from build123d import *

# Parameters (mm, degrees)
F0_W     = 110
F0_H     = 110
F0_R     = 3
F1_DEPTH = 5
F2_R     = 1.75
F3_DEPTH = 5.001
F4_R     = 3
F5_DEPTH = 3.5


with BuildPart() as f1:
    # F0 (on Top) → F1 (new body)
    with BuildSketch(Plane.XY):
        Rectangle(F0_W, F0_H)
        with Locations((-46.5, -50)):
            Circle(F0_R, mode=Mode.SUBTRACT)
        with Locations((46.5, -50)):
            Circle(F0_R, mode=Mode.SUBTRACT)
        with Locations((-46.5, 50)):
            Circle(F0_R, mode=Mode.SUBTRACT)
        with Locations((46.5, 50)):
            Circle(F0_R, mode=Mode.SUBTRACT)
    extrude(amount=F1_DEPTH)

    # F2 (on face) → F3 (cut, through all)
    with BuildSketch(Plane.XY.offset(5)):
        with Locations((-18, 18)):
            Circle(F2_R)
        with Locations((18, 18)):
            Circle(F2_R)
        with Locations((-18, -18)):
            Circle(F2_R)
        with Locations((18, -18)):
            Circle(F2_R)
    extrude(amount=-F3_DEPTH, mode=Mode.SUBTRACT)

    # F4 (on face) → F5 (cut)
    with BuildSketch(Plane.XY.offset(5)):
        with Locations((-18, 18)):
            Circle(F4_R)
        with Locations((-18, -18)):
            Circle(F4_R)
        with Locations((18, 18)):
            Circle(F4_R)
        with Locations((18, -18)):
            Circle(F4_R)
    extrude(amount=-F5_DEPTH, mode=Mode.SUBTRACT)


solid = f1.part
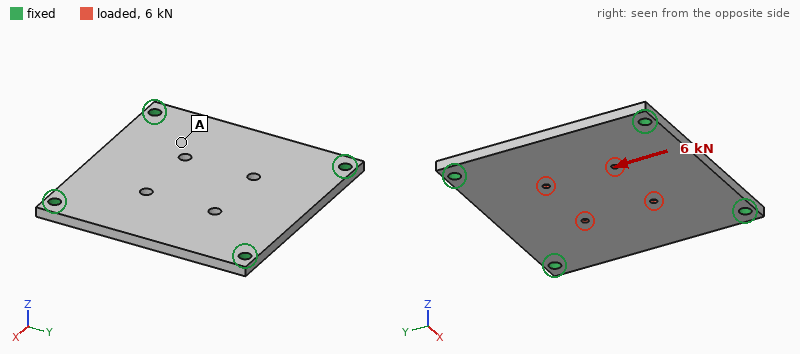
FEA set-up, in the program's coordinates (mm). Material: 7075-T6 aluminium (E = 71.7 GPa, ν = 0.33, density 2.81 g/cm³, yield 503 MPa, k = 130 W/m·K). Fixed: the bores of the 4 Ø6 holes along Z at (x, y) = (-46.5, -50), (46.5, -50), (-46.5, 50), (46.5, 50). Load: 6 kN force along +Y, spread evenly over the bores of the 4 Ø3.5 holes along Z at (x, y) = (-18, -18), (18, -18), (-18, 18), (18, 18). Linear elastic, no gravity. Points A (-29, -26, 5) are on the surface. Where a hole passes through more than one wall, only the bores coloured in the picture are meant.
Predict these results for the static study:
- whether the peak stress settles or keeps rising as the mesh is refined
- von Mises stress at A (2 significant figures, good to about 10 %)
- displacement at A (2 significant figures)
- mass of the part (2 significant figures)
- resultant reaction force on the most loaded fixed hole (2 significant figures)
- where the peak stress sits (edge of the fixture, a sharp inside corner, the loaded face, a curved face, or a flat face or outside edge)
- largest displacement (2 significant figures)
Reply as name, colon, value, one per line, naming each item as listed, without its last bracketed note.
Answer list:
whether the peak stress settles or keeps rising as the mesh is refined: keeps rising
von Mises stress at A: 8.7 MPa
displacement at A: 8.8 µm
mass of the part: 170 g
resultant reaction force on the most loaded fixed hole: 1.7 kN
where the peak stress sits: a sharp inside corner
largest displacement: 17 µm
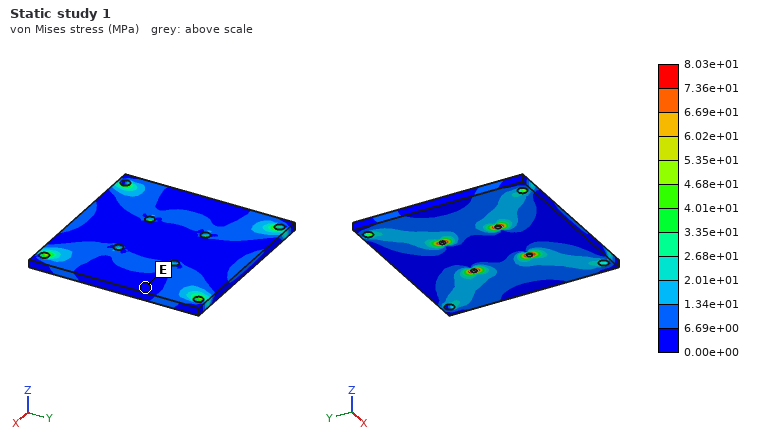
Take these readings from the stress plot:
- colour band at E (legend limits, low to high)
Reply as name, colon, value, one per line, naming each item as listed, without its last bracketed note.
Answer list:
colour band at E: 0.00e+00 to 6.69e+00 MPa
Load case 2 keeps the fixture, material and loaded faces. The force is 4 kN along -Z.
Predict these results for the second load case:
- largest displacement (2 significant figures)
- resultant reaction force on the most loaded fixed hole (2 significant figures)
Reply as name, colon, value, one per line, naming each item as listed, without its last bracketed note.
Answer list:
largest displacement: 0.49 mm
resultant reaction force on the most loaded fixed hole: 1.0 kN
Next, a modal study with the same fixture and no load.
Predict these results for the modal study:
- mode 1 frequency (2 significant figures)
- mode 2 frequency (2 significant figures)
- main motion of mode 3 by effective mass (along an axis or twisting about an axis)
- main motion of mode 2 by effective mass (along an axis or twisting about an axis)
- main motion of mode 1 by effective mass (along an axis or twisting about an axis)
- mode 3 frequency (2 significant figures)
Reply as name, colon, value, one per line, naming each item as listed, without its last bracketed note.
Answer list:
mode 1 frequency: 1800 Hz
mode 2 frequency: 3000 Hz
main motion of mode 3 by effective mass: twisting about X
main motion of mode 2 by effective mass: twisting about Y
main motion of mode 1 by effective mass: along Z
mode 3 frequency: 3300 Hz
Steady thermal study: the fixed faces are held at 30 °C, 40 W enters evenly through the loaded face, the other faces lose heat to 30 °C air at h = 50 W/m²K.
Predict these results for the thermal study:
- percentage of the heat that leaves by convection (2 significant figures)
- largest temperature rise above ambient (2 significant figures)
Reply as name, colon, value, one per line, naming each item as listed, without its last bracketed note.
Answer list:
percentage of the heat that leaves by convection: 30 %
largest temperature rise above ambient: 22 K
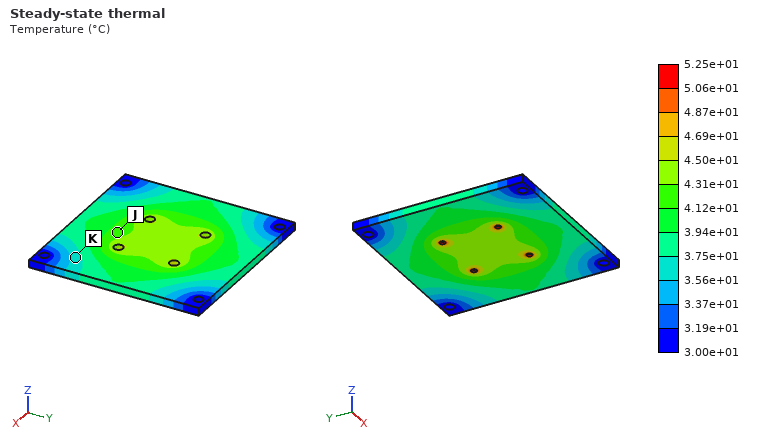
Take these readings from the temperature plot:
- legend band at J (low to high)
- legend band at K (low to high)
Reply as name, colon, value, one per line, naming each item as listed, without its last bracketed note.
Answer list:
legend band at J: 4.12e+01 to 4.31e+01 °C
legend band at K: 3.56e+01 to 3.75e+01 °C
